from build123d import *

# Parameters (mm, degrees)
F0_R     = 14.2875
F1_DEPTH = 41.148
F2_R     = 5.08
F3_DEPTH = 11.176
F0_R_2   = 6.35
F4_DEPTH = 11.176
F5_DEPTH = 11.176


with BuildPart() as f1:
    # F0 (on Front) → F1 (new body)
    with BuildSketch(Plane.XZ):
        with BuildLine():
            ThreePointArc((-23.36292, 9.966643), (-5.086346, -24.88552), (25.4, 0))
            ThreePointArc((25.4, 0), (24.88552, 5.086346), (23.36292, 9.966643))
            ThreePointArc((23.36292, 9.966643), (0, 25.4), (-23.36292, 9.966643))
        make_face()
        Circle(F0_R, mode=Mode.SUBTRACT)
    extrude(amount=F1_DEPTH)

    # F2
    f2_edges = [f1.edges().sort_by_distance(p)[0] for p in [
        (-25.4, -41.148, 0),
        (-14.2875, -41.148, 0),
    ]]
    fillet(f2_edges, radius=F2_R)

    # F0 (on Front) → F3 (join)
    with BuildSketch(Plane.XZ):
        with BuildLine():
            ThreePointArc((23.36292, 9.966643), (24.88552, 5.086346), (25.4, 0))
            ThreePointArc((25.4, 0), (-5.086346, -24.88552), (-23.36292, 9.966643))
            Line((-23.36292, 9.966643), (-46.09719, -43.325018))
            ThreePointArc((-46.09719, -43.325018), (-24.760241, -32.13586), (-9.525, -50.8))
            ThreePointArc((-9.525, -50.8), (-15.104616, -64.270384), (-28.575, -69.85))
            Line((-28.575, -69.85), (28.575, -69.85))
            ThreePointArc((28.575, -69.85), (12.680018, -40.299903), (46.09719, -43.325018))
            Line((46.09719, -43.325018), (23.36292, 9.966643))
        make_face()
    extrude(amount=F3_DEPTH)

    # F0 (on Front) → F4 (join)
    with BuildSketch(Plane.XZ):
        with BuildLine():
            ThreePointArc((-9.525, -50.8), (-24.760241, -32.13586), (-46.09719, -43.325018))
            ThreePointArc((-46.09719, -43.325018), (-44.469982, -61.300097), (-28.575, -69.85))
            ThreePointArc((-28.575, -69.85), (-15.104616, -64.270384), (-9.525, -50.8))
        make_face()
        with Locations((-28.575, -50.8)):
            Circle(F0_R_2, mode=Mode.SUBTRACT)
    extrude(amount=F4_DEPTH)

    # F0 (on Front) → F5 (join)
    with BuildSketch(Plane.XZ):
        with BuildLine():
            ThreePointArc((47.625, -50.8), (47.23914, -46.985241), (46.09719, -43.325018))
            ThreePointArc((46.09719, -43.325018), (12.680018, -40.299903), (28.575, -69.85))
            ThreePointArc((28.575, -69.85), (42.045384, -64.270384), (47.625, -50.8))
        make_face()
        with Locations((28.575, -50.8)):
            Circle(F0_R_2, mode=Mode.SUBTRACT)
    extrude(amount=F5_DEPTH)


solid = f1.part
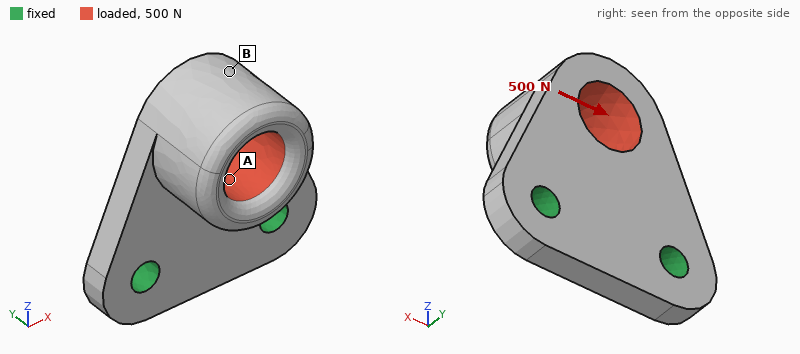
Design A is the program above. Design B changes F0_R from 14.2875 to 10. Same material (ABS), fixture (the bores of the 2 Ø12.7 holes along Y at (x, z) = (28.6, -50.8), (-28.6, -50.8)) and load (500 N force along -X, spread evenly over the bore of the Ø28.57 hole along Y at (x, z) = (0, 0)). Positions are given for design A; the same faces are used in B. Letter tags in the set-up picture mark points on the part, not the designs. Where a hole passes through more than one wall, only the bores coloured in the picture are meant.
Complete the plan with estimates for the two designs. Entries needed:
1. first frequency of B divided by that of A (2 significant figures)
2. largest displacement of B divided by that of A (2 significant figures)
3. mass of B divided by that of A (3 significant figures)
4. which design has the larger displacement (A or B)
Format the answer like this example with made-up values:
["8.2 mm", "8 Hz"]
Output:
["0.91", "0.91", "1.13", "A"]
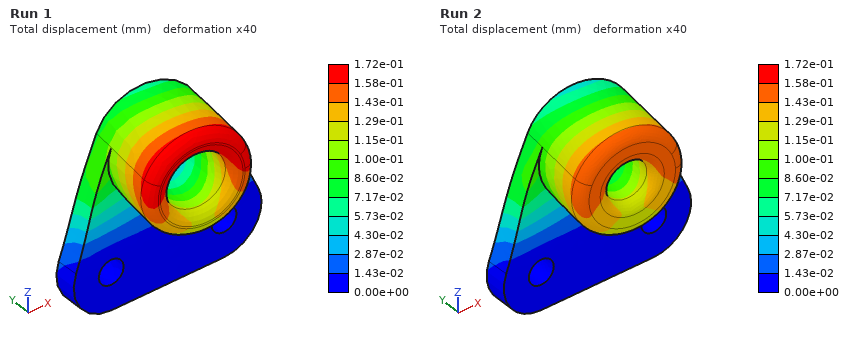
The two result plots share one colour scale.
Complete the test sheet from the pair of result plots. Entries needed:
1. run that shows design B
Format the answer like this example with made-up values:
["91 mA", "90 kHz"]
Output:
["Run 2"]
